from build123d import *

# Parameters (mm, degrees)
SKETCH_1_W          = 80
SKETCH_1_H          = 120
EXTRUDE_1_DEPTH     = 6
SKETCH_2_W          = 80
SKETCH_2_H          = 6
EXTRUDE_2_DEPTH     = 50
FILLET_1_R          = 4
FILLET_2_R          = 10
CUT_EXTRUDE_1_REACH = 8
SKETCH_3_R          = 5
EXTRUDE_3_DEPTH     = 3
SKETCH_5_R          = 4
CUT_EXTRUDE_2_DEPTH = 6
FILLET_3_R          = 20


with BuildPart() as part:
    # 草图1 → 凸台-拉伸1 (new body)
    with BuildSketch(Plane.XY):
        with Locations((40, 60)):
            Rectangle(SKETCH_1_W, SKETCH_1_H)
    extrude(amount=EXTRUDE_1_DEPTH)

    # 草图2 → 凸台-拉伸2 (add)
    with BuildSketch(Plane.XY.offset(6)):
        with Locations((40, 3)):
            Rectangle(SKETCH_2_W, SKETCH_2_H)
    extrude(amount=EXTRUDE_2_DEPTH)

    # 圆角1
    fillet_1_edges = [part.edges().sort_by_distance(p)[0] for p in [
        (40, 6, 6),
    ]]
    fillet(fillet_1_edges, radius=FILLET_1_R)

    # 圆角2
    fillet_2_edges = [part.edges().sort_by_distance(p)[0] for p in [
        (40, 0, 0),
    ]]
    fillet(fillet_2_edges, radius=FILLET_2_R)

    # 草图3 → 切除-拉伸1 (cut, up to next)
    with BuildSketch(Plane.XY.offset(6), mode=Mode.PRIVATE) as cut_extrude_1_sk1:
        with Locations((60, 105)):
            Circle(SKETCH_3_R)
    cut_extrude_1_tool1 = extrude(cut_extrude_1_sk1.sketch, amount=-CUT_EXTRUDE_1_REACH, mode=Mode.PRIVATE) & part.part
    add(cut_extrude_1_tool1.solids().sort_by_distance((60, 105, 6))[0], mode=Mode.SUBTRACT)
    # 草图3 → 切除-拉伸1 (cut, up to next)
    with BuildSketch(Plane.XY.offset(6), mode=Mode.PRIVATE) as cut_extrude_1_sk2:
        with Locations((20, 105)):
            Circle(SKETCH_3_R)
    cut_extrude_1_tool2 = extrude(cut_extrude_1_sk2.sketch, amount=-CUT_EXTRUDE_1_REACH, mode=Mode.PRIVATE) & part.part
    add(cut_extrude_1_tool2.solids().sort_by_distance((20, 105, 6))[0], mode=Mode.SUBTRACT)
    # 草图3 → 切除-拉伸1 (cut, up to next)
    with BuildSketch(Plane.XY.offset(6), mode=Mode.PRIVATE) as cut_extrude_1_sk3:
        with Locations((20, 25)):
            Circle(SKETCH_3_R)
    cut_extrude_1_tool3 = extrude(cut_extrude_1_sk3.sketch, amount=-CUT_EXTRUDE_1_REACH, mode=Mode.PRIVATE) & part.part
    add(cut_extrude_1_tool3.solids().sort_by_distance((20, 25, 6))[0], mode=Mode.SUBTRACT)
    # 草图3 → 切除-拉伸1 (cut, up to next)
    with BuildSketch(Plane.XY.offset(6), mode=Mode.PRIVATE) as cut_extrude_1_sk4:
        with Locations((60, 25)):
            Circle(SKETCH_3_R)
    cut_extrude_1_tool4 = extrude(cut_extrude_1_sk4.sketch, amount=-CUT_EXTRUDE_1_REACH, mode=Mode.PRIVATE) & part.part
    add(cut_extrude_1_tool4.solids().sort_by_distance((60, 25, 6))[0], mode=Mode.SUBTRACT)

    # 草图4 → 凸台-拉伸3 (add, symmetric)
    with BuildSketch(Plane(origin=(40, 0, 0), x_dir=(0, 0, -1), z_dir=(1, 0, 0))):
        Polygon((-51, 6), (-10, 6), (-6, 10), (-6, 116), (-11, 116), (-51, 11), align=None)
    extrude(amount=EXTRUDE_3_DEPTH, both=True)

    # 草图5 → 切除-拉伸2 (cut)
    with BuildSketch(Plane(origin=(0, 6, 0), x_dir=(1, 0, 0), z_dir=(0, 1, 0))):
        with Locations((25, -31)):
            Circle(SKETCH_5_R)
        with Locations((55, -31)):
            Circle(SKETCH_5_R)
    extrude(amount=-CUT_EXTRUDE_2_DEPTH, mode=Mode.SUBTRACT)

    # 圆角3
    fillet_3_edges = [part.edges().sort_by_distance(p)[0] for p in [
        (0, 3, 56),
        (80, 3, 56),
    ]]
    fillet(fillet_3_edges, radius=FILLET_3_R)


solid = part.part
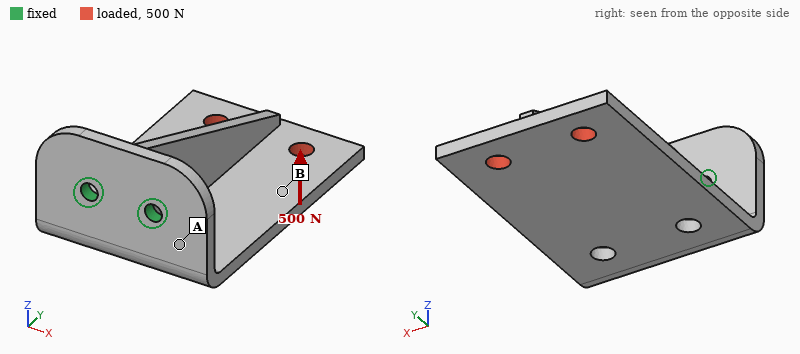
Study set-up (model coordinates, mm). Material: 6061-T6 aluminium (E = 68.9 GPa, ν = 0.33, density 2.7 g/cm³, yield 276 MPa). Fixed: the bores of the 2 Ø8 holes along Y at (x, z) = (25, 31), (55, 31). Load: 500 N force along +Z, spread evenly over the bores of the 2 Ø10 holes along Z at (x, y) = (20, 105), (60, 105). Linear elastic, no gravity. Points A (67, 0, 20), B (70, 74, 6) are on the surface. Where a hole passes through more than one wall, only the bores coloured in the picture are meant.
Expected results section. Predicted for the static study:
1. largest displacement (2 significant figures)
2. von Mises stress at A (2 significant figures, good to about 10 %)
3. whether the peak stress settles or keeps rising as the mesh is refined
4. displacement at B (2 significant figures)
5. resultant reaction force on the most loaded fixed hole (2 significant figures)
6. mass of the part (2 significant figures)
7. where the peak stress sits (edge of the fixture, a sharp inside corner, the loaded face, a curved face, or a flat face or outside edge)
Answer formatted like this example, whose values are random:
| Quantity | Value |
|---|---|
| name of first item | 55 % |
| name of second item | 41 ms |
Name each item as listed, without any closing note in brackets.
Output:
| Quantity | Value |
|---|---|
| largest displacement | 0.36 mm |
| von Mises stress at A | 22 MPa |
| whether the peak stress settles or keeps rising as the mesh is refined | keeps rising |
| displacement at B | 0.20 mm |
| resultant reaction force on the most loaded fixed hole | 260 N |
| mass of the part | 250 g |
| where the peak stress sits | edge of the fixture |
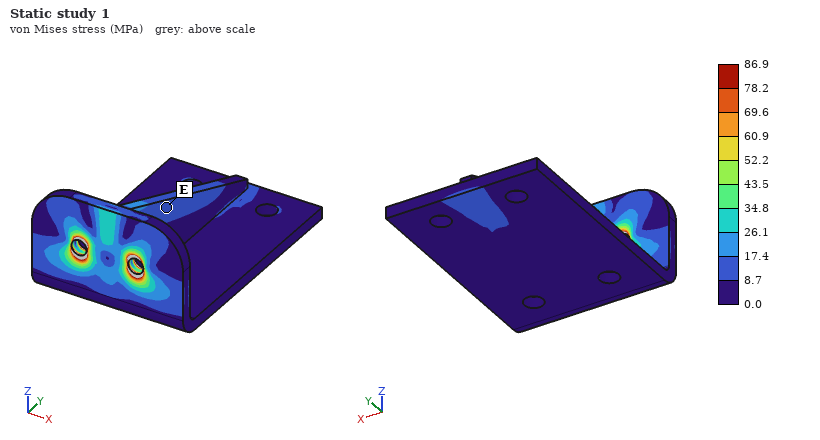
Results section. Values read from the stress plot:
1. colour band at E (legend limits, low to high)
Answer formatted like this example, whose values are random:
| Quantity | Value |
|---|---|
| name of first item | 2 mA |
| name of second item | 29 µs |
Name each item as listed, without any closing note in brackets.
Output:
| Quantity | Value |
|---|---|
| colour band at E | 8.7 to 17.4 MPa |
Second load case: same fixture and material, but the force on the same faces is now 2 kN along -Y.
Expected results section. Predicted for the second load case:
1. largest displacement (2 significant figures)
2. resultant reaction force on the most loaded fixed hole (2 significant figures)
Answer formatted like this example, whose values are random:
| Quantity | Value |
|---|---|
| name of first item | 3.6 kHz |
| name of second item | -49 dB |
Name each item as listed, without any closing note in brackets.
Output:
| Quantity | Value |
|---|---|
| largest displacement | 0.33 mm |
| resultant reaction force on the most loaded fixed hole | 1.0 kN |
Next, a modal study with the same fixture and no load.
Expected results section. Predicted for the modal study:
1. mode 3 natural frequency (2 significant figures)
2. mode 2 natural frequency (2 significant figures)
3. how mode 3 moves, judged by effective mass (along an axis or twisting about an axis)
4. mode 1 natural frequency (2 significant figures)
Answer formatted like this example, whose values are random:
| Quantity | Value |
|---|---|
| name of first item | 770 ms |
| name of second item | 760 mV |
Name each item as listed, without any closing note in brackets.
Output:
| Quantity | Value |
|---|---|
| mode 3 natural frequency | 1300 Hz |
| mode 2 natural frequency | 730 Hz |
| how mode 3 moves, judged by effective mass | twisting about Y |
| mode 1 natural frequency | 730 Hz |
